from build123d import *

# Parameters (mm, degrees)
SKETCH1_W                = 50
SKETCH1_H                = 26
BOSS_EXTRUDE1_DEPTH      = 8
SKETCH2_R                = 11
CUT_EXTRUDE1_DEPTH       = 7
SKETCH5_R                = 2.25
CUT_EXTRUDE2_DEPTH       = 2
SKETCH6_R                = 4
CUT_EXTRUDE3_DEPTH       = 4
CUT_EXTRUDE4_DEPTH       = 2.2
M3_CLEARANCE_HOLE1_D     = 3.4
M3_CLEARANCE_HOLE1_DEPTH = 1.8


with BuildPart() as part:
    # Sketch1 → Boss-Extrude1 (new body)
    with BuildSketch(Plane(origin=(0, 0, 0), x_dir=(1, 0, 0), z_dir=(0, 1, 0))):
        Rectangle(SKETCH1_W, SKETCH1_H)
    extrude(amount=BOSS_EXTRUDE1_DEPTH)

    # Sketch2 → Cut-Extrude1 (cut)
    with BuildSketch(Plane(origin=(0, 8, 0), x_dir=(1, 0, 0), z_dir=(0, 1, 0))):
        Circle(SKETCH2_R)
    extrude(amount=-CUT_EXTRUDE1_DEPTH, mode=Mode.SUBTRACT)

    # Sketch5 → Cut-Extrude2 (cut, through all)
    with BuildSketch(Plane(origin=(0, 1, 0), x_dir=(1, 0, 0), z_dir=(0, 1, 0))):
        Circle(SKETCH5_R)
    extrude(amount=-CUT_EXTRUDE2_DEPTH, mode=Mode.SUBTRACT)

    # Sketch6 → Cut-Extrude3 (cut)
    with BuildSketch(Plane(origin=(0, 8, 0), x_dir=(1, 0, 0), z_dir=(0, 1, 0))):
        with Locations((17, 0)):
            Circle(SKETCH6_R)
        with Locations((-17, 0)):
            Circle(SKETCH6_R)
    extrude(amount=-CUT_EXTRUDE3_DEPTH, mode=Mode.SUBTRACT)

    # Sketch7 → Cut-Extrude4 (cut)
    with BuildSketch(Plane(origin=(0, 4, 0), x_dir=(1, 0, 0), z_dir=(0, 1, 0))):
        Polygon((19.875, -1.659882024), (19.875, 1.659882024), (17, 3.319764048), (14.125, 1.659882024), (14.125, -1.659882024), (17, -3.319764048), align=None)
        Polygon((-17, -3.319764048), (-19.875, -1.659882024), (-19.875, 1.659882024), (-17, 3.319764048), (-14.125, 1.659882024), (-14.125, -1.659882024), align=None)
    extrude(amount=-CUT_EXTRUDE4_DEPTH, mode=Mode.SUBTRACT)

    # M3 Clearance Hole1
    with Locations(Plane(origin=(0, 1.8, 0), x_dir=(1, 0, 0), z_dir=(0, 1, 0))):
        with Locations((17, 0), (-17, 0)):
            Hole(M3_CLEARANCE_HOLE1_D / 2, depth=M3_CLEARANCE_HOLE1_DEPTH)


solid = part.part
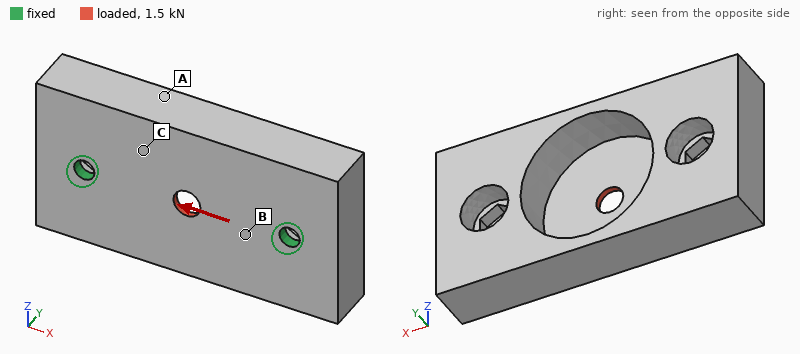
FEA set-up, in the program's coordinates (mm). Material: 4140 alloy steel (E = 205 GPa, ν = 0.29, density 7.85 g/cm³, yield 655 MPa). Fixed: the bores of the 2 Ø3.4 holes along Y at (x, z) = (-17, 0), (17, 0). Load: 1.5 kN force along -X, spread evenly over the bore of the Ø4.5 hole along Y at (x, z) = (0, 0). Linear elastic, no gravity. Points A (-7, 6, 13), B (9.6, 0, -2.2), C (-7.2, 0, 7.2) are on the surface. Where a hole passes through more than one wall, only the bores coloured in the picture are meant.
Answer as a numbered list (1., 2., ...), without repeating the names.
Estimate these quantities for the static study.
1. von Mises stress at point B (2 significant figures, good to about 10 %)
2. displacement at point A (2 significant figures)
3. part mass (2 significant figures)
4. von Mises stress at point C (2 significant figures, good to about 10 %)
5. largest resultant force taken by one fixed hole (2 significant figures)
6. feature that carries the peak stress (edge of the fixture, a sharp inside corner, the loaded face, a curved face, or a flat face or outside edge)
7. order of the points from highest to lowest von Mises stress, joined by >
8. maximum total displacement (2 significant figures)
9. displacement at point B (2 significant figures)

1. 47 MPa
2. 0.92 µm
3. 56 g
4. 22 MPa
5. 750 N
6. the loaded face
7. B > C > A
8. 4.3 µm
9. 1.5 µm
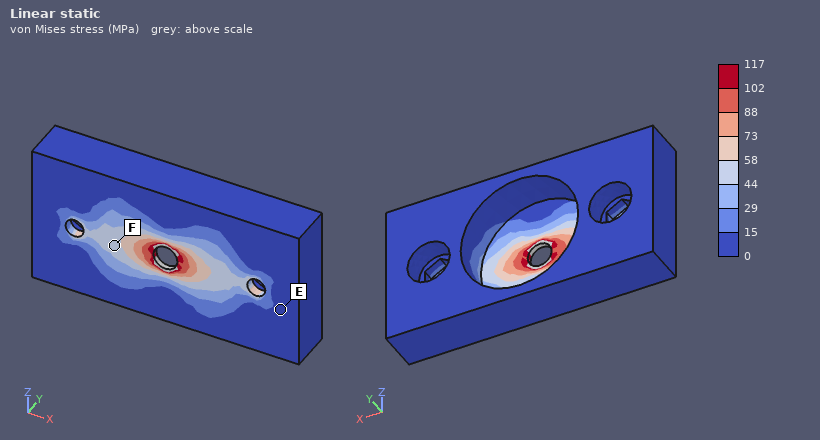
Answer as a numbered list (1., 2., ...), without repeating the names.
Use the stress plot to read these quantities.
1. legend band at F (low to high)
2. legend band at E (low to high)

1. 44 to 58 MPa
2. 0 to 15 MPa
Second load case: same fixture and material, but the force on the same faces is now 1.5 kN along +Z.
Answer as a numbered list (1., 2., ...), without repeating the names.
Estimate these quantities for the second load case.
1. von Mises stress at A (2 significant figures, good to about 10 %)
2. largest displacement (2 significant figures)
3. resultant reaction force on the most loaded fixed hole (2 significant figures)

1. 17 MPa
2. 6.4 µm
3. 750 N
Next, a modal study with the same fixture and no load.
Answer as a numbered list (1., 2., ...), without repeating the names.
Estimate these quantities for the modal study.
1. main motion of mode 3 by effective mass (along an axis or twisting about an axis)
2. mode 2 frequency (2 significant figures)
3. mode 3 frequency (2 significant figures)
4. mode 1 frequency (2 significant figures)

1. along Y
2. 11 kHz
3. 13 kHz
4. 5200 Hz
